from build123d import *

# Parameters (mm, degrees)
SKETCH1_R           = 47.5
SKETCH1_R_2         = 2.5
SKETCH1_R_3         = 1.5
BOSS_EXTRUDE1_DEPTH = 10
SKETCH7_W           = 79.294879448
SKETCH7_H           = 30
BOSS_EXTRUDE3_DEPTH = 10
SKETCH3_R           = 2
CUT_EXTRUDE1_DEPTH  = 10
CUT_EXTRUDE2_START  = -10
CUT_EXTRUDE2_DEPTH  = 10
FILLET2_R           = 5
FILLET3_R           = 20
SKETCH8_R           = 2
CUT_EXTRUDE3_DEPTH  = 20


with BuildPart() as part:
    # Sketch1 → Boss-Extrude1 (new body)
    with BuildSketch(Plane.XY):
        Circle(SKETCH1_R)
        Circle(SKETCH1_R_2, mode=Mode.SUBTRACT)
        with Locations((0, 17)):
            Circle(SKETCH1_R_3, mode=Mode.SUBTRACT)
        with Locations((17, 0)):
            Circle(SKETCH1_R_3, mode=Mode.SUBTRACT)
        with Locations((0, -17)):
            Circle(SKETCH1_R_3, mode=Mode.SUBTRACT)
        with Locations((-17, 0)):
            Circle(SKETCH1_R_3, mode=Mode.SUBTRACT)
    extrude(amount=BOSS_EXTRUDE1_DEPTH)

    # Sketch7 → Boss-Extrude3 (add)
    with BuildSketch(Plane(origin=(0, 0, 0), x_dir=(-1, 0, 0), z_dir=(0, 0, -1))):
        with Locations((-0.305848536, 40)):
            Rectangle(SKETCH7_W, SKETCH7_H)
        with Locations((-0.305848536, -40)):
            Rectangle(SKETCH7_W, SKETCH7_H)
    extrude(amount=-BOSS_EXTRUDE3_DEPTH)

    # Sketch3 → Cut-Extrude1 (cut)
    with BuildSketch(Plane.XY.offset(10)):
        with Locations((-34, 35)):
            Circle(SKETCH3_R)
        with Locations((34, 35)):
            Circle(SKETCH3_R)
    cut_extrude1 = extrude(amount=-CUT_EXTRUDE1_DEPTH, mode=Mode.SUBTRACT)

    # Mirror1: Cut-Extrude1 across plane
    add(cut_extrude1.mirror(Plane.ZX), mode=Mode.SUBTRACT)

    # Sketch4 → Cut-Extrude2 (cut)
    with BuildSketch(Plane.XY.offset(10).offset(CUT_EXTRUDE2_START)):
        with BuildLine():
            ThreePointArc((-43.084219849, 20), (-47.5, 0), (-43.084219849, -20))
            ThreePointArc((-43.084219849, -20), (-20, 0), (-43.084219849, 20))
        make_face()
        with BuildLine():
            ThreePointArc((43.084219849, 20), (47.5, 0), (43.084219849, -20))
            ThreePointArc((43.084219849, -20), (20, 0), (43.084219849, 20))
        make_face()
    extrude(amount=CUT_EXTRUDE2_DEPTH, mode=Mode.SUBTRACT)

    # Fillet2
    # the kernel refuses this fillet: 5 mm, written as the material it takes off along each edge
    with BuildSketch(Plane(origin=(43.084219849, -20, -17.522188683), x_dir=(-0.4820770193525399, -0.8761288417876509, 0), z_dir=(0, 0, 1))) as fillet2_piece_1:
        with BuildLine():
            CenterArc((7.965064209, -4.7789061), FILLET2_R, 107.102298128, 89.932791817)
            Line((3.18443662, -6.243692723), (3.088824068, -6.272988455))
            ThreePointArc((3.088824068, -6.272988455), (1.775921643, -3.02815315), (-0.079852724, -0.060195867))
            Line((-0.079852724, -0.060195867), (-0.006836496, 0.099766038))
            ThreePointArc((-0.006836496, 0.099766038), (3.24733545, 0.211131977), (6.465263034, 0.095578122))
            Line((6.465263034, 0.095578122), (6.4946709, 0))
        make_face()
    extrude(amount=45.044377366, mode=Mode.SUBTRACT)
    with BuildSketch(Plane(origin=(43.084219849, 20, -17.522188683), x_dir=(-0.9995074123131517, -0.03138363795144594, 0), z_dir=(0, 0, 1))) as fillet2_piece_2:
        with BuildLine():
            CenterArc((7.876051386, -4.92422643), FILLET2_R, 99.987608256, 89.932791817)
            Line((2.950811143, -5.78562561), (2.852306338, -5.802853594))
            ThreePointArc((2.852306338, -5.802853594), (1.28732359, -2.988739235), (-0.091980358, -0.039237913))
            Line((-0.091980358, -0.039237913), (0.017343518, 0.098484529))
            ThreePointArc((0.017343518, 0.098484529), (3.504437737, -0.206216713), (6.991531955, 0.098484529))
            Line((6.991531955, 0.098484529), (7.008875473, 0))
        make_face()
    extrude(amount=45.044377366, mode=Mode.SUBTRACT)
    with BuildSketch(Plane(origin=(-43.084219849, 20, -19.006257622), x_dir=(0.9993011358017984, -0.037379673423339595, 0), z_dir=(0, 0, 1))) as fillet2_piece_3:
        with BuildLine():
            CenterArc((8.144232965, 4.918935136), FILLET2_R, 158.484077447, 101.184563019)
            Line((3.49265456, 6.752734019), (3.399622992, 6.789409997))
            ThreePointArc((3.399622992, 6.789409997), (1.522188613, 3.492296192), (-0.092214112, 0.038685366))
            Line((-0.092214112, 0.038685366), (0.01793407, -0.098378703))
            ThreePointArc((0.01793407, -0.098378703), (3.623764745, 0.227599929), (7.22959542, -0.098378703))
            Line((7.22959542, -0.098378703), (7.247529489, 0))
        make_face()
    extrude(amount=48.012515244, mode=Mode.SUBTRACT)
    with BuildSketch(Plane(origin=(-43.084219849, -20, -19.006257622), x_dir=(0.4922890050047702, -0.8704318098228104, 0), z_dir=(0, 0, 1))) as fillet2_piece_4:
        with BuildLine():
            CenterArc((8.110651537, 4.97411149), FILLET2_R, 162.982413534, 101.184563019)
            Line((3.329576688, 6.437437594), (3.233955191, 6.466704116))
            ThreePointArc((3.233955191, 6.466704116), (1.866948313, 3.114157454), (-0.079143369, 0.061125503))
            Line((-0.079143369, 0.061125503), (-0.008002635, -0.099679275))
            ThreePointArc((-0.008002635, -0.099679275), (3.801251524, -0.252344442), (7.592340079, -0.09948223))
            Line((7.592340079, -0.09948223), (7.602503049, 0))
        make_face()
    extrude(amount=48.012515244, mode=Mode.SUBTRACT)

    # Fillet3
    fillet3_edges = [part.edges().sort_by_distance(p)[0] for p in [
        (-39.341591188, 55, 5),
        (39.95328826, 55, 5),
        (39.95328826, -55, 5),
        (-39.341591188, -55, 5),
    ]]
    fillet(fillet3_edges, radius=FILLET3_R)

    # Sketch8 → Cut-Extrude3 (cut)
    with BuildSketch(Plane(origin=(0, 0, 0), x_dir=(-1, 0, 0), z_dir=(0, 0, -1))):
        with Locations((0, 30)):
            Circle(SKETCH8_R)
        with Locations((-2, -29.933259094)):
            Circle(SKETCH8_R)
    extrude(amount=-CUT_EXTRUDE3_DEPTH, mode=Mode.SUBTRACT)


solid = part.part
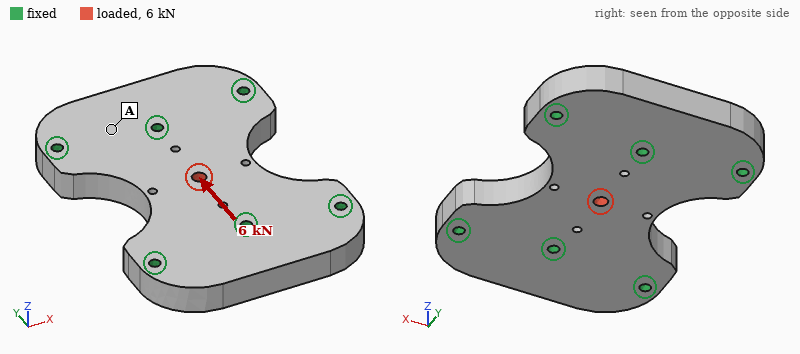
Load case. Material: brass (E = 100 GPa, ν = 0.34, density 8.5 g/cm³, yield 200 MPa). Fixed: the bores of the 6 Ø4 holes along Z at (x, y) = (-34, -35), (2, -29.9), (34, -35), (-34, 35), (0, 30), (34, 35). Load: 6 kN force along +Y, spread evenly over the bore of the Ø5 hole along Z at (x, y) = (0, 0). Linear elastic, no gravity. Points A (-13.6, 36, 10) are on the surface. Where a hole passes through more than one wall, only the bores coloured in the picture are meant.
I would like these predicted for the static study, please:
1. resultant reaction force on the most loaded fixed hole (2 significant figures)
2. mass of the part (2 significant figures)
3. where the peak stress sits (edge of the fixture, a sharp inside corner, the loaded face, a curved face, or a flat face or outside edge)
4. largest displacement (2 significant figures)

1.8 kN
600 g
the loaded face
4.8 µm
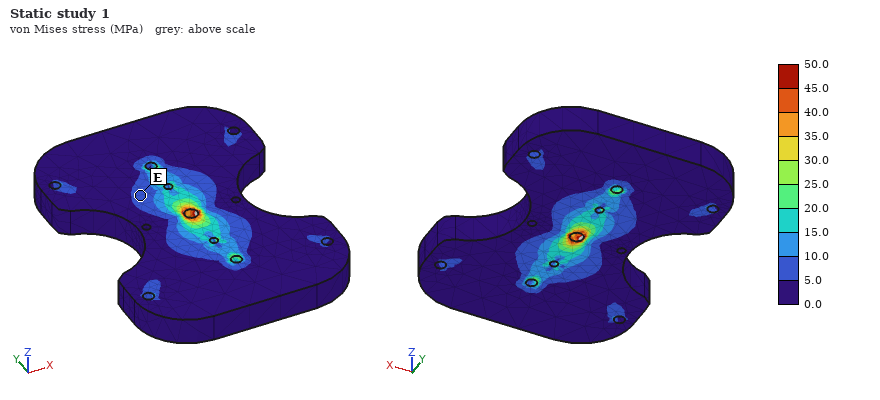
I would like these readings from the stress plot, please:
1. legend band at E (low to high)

5.0 to 10.0 MPa
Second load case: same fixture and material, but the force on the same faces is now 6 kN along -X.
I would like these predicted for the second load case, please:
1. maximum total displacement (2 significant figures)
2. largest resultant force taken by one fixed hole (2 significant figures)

7.4 µm
1.5 kN
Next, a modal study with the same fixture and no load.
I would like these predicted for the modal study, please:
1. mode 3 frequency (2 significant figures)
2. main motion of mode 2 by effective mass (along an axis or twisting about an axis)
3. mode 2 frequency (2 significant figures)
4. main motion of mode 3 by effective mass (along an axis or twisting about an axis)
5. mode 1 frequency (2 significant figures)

8700 Hz
twisting about X
8000 Hz
along Z
6500 Hz
